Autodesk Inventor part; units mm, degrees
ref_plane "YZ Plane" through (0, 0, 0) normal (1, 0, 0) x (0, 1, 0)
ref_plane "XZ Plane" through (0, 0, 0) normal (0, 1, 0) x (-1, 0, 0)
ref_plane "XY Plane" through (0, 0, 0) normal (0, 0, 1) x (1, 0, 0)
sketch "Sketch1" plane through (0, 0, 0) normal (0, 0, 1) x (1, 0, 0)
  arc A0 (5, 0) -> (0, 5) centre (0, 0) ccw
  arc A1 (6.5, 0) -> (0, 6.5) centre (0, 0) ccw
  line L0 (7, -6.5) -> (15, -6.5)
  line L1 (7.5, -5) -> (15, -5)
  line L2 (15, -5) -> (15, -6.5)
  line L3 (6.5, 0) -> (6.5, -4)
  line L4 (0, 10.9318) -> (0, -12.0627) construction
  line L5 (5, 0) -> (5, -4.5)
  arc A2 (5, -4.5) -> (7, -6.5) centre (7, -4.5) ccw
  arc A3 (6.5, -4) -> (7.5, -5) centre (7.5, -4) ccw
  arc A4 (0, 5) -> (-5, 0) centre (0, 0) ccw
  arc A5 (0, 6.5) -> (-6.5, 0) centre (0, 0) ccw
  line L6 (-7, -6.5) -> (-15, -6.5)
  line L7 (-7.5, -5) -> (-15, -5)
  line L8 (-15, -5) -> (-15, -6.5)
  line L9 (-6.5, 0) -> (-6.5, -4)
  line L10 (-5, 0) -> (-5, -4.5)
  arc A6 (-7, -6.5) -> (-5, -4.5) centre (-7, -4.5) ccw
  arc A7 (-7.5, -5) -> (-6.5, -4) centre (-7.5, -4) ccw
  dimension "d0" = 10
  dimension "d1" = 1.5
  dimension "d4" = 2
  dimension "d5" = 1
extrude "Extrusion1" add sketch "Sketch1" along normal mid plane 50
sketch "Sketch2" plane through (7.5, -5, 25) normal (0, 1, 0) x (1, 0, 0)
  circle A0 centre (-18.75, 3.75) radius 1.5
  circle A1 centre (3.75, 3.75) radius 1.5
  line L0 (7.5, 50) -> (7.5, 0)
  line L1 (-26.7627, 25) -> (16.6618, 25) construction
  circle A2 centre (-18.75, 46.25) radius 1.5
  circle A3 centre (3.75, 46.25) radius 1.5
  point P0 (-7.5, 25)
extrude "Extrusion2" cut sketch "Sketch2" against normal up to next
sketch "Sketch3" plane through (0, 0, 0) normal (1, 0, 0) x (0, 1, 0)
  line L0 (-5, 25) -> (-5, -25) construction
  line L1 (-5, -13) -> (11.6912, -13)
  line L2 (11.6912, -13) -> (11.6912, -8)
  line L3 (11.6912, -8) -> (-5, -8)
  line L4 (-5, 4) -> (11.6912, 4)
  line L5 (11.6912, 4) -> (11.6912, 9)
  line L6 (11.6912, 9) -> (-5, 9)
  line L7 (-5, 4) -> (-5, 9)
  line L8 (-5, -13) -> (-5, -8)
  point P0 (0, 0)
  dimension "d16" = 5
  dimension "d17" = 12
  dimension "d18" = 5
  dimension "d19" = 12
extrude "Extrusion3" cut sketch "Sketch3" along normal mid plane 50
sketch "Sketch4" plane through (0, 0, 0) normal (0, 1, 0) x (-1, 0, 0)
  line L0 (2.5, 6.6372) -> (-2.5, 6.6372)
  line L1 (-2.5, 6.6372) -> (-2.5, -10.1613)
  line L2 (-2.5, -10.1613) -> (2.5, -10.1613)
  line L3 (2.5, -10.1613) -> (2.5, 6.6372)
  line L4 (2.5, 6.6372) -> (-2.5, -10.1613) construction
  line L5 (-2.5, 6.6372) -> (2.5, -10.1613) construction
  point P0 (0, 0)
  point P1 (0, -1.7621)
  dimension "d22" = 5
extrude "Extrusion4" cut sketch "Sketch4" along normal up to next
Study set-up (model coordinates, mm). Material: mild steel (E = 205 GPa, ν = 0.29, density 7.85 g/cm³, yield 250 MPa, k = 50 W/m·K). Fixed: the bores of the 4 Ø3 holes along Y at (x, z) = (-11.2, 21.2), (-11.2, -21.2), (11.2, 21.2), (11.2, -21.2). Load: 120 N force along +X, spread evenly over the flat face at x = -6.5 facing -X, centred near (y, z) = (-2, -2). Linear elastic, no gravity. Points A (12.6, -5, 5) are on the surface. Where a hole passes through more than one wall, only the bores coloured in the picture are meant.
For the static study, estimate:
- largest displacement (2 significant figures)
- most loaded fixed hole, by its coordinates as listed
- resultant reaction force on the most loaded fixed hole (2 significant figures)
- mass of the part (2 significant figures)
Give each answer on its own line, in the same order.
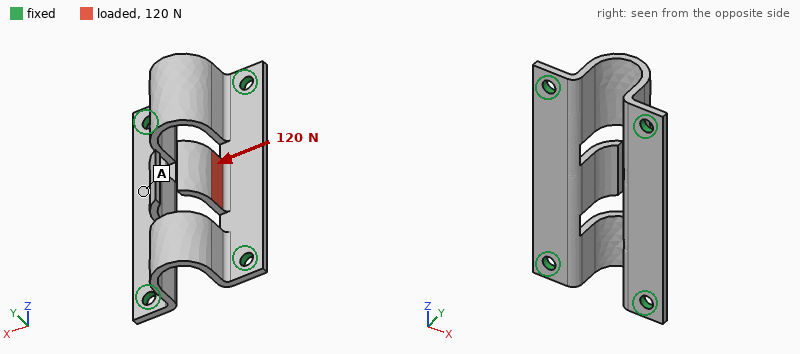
67 µm
(-11.2, -21.2)
64 N
23 g
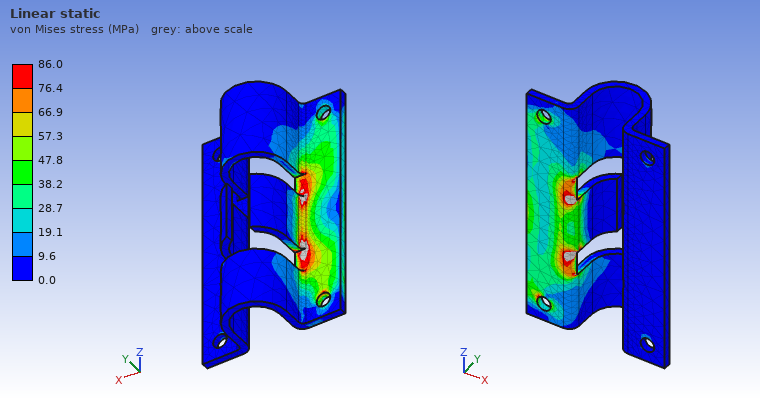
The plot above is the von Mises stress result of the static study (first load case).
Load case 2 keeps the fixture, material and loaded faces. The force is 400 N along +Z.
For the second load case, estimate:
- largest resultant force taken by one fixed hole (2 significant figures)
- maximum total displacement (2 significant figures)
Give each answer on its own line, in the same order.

250 N
42 µm
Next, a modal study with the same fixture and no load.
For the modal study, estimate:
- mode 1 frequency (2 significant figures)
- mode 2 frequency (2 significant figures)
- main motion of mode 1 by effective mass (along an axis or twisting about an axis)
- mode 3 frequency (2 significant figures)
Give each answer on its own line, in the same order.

3800 Hz
4500 Hz
along Y
4800 Hz
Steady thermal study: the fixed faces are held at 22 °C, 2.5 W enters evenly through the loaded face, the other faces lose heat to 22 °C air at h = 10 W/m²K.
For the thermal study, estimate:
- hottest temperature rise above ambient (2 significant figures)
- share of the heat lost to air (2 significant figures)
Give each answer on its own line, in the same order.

37 K
11 %
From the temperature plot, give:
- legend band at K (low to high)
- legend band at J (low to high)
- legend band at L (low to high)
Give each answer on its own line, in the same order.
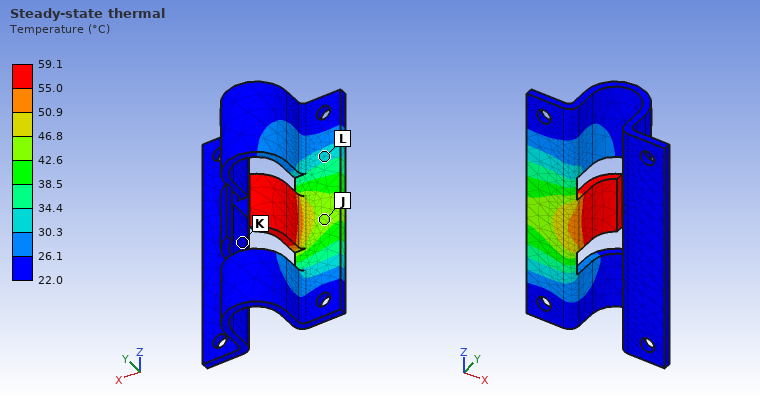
22.0 to 26.1 °C
42.6 to 46.8 °C
30.3 to 34.4 °C
